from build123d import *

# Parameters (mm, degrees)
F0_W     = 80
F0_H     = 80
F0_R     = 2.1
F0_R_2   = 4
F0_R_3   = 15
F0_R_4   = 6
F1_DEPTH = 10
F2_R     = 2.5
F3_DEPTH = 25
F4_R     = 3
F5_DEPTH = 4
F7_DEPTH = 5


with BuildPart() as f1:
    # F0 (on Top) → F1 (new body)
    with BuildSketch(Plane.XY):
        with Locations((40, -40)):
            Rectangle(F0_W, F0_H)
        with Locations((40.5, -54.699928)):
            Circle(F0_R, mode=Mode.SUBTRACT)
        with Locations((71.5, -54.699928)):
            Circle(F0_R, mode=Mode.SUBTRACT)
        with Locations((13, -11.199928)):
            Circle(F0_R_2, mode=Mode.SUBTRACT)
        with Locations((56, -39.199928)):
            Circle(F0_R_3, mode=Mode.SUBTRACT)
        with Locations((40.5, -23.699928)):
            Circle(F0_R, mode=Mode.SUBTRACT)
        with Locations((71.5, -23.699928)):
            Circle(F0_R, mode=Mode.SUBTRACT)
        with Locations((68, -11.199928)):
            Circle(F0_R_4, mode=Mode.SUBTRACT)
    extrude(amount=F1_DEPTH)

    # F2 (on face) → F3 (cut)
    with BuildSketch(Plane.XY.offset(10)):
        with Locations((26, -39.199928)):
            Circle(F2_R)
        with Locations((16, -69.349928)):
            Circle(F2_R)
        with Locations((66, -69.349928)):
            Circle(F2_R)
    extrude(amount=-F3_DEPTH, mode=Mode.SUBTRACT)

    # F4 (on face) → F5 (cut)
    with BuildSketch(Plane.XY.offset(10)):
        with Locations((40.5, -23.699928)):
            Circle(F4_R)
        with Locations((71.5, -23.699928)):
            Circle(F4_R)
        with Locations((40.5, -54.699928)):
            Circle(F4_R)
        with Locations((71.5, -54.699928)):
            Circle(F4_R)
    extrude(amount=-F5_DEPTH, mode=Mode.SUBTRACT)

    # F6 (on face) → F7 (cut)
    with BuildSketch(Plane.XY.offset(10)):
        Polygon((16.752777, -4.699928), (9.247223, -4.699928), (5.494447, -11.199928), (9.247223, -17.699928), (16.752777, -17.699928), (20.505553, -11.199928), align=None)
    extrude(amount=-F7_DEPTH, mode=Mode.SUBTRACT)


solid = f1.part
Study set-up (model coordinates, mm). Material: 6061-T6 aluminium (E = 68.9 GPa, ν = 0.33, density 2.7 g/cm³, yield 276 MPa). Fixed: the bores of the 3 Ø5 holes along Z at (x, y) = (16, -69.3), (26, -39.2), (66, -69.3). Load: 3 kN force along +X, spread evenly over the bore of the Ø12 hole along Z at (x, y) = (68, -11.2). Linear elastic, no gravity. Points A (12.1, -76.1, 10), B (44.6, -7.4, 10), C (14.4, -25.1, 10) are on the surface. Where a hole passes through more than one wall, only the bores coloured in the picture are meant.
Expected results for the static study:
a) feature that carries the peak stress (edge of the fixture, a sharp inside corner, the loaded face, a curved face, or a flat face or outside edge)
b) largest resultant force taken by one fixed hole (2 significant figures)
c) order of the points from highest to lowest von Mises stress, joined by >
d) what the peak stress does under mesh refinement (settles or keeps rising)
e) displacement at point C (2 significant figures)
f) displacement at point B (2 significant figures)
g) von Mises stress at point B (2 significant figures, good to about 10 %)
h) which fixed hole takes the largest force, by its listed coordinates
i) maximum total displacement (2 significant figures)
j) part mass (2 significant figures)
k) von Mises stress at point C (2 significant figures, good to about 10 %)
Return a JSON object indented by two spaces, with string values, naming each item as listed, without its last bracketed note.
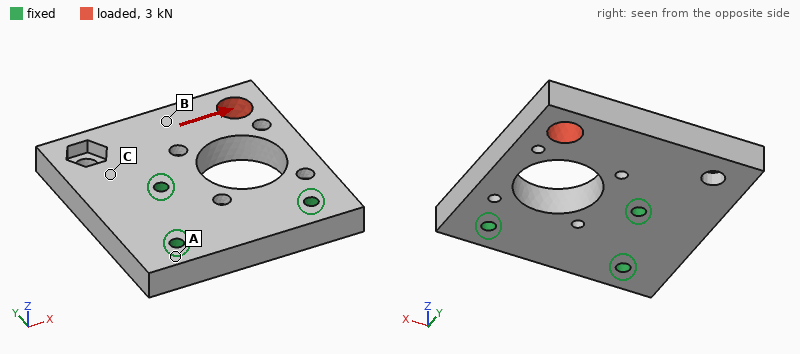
{
  "feature that carries the peak stress": "edge of the fixture",
  "largest resultant force taken by one fixed hole": "3.5 kN",
  "order of the points from highest to lowest von Mises stress, joined by >": "C > B > A",
  "what the peak stress does under mesh refinement": "keeps rising",
  "displacement at point C": "8.7 µm",
  "displacement at point B": "20 µm",
  "von Mises stress at point B": "6.7 MPa",
  "which fixed hole takes the largest force, by its listed coordinates": "(26, -39.2)",
  "maximum total displacement": "28 µm",
  "part mass": "140 g",
  "von Mises stress at point C": "11 MPa"
}
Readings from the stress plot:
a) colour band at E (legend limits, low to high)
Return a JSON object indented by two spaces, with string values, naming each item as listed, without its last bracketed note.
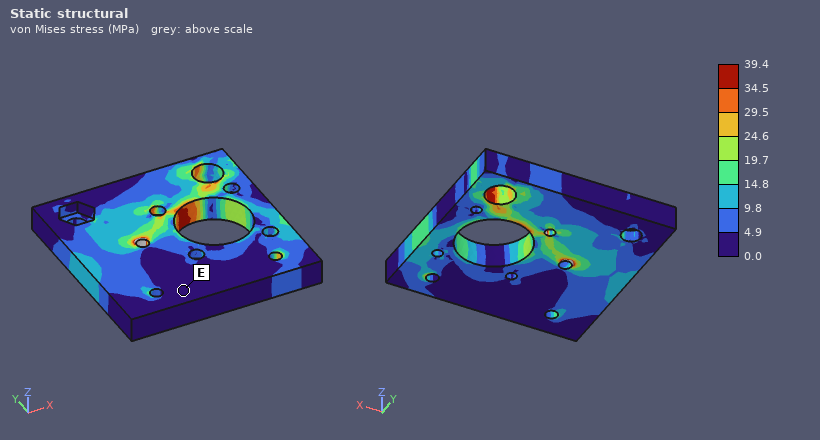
{
  "colour band at E": "0.0 to 4.9 MPa"
}
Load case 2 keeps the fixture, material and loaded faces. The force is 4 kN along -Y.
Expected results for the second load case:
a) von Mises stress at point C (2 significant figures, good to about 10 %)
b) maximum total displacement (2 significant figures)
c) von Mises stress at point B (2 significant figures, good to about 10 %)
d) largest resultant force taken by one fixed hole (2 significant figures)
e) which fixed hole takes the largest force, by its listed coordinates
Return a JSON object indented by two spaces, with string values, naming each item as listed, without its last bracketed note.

{
  "von Mises stress at point C": "8.1 MPa",
  "maximum total displacement": "34 µm",
  "von Mises stress at point B": "5.8 MPa",
  "largest resultant force taken by one fixed hole": "3.2 kN",
  "which fixed hole takes the largest force, by its listed coordinates": "(66, -69.3)"
}
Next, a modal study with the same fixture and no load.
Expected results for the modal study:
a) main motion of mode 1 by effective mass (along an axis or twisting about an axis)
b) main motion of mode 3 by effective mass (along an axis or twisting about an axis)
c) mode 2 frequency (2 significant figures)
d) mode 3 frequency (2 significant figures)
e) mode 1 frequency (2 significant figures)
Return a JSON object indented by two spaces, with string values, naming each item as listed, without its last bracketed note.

{
  "main motion of mode 1 by effective mass": "along Z",
  "main motion of mode 3 by effective mass": "along X",
  "mode 2 frequency": "4900 Hz",
  "mode 3 frequency": "8200 Hz",
  "mode 1 frequency": "2700 Hz"
}
